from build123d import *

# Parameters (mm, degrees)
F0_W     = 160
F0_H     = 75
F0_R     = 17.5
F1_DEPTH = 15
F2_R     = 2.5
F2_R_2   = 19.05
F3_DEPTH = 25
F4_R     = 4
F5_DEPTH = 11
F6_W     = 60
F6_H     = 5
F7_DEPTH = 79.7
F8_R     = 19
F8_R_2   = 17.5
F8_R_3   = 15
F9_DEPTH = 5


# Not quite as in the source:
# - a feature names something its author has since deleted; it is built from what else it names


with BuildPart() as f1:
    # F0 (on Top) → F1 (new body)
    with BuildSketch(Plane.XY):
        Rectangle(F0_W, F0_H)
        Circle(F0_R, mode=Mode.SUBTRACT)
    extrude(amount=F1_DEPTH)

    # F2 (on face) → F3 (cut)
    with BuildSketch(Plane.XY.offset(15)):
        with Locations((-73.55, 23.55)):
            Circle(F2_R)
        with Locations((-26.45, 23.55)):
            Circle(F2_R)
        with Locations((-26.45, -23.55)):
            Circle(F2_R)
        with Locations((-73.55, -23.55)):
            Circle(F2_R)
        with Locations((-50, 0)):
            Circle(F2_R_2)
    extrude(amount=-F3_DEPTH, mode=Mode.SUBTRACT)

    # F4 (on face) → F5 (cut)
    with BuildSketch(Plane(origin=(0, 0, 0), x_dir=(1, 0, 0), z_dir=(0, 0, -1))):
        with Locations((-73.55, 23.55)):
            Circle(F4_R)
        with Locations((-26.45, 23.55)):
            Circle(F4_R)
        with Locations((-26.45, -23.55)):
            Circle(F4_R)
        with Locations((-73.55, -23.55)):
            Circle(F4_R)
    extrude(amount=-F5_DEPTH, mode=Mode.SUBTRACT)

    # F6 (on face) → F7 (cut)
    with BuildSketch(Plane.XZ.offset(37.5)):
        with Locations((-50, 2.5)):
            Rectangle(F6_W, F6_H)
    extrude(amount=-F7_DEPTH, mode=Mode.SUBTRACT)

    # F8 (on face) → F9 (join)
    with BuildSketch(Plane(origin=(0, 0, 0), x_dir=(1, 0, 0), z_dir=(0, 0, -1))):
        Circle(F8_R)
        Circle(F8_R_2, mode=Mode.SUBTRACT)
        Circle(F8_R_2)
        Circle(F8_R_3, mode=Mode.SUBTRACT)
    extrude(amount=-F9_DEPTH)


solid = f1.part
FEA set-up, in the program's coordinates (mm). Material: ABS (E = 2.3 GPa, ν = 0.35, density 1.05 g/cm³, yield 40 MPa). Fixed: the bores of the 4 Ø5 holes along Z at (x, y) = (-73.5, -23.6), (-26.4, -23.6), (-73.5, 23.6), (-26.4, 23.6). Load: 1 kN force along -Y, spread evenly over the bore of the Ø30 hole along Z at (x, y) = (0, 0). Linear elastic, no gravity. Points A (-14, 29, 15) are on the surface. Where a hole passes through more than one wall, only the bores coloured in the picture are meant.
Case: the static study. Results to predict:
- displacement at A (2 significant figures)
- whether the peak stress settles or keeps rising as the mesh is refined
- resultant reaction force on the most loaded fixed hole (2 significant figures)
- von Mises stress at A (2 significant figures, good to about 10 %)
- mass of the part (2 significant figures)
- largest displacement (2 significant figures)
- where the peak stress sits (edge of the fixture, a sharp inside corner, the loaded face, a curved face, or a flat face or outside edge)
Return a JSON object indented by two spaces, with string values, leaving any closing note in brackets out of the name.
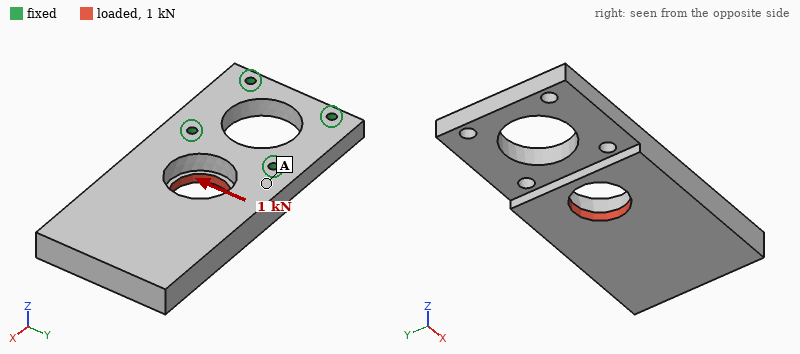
{
  "displacement at A": "0.065 mm",
  "whether the peak stress settles or keeps rising as the mesh is refined": "keeps rising",
  "resultant reaction force on the most loaded fixed hole": "670 N",
  "von Mises stress at A": "1.7 MPa",
  "mass of the part": "140 g",
  "largest displacement": "0.28 mm",
  "where the peak stress sits": "edge of the fixture"
}
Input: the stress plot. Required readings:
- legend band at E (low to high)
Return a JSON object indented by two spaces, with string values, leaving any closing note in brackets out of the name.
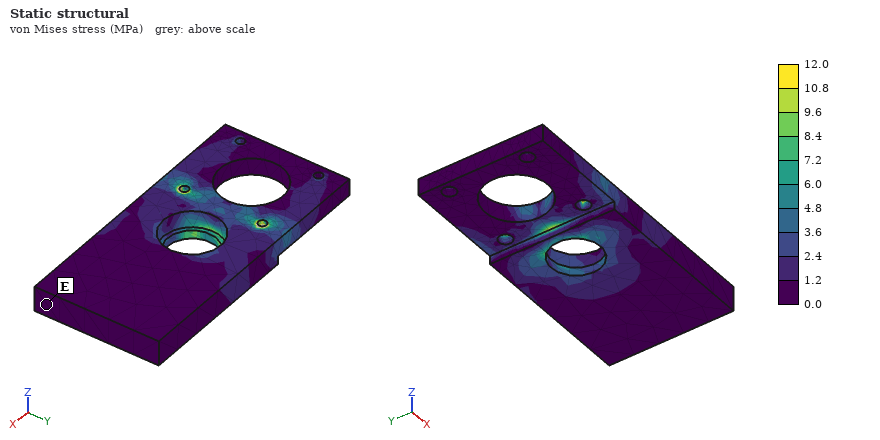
{
  "legend band at E": "0.0 to 1.2 MPa"
}
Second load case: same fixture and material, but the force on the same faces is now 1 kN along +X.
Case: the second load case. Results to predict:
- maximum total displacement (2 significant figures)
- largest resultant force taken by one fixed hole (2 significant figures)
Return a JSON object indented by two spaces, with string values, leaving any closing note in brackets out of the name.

{
  "maximum total displacement": "1.9 mm",
  "largest resultant force taken by one fixed hole": "270 N"
}
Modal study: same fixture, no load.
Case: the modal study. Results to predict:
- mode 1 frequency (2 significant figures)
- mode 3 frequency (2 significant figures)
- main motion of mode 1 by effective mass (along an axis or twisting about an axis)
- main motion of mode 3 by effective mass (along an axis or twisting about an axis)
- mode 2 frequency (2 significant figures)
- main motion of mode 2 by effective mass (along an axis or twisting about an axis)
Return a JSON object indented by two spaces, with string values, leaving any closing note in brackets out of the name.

{
  "mode 1 frequency": "160 Hz",
  "mode 3 frequency": "780 Hz",
  "main motion of mode 1 by effective mass": "along Z",
  "main motion of mode 3 by effective mass": "along Y",
  "mode 2 frequency": "620 Hz",
  "main motion of mode 2 by effective mass": "along Y"
}
